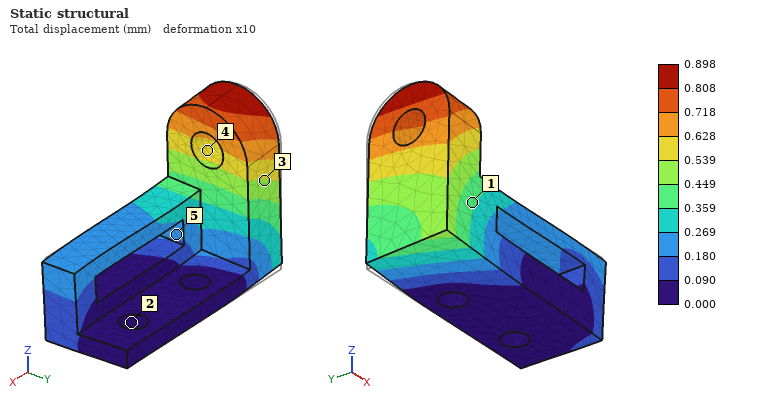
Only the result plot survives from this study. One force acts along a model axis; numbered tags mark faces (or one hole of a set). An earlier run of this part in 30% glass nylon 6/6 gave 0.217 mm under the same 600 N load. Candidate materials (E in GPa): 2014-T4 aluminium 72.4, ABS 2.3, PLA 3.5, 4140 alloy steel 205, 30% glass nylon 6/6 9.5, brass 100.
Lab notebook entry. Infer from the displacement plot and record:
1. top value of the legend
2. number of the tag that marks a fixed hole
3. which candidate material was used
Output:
0.898 mm
2
ABS
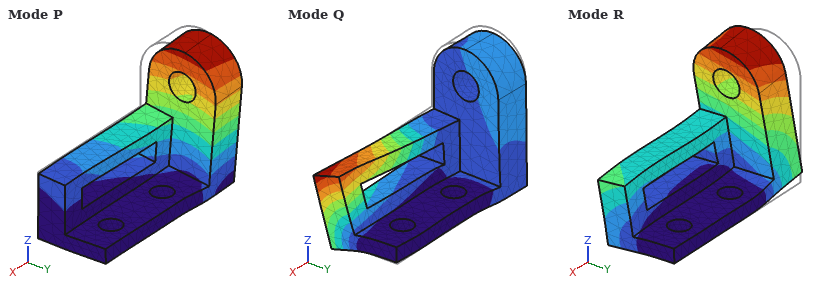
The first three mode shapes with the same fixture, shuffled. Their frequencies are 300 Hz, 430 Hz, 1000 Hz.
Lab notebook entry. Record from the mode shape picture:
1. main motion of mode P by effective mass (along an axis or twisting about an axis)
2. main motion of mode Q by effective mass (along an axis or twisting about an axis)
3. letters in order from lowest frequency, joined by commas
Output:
along Y
along Z
P, R, Q
